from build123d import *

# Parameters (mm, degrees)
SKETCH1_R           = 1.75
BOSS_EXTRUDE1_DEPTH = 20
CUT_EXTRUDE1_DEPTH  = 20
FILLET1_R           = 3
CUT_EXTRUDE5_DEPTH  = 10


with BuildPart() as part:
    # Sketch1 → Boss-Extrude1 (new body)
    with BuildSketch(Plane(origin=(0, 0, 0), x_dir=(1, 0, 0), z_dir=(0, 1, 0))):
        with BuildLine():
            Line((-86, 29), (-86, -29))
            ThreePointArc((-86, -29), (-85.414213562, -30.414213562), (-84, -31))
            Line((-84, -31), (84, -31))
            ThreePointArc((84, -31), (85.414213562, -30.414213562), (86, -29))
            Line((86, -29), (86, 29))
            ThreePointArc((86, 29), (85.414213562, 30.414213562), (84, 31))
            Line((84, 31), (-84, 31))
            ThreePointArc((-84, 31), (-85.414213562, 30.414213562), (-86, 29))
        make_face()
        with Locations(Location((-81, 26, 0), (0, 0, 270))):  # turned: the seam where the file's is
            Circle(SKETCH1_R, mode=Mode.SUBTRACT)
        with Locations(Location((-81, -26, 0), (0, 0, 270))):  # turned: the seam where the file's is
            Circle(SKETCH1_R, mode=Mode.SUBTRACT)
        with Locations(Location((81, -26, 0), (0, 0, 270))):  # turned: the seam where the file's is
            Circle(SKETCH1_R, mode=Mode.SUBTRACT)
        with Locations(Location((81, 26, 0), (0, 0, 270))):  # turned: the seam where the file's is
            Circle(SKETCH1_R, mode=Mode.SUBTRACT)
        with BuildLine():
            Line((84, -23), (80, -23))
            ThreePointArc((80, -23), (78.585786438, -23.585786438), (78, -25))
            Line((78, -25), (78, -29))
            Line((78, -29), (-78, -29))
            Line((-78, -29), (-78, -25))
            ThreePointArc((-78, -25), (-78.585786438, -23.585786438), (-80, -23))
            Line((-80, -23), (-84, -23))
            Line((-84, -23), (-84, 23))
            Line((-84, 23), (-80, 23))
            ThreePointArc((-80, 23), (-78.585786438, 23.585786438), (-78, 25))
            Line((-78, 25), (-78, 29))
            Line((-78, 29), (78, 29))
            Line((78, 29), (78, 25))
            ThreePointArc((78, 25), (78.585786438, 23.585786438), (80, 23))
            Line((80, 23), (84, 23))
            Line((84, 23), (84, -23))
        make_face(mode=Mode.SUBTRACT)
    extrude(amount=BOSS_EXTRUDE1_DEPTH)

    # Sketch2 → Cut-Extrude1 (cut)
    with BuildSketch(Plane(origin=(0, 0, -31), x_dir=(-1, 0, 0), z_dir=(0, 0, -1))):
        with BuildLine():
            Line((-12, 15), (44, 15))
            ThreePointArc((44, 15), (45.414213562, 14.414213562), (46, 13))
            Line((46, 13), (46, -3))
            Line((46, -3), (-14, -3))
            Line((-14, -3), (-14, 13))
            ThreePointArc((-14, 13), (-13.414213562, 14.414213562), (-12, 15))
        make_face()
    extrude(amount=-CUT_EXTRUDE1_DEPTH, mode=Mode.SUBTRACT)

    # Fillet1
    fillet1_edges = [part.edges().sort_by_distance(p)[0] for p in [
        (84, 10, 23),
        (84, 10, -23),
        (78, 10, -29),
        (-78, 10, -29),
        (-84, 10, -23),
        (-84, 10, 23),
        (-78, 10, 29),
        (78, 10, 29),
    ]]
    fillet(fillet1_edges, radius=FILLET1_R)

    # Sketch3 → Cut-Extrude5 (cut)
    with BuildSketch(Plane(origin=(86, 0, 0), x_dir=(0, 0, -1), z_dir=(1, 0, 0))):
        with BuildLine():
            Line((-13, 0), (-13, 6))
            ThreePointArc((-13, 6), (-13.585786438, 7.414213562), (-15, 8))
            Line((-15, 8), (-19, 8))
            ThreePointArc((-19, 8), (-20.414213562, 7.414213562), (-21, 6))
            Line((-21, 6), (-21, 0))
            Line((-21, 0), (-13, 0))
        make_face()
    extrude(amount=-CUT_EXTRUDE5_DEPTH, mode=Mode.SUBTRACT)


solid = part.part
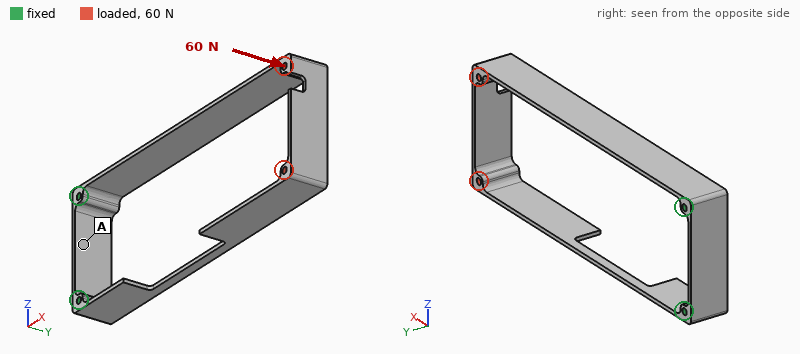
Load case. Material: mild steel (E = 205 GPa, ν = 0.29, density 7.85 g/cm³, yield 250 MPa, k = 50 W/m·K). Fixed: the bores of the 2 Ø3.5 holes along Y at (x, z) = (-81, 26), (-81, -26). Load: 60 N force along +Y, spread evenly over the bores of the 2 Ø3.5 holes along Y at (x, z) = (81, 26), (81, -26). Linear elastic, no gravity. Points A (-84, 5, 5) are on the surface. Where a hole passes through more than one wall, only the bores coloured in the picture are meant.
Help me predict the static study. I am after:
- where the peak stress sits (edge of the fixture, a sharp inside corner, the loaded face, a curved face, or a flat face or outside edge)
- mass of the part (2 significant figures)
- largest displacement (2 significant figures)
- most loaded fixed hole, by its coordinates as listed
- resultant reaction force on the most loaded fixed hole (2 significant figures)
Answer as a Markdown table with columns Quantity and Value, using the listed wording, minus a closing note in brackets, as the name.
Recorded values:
| Quantity | Value |
|---|---|
| where the peak stress sits | a curved face |
| mass of the part | 150 g |
| largest displacement | 1.4 mm |
| most loaded fixed hole, by its coordinates as listed | (-81, 26) |
| resultant reaction force on the most loaded fixed hole | 47 N |
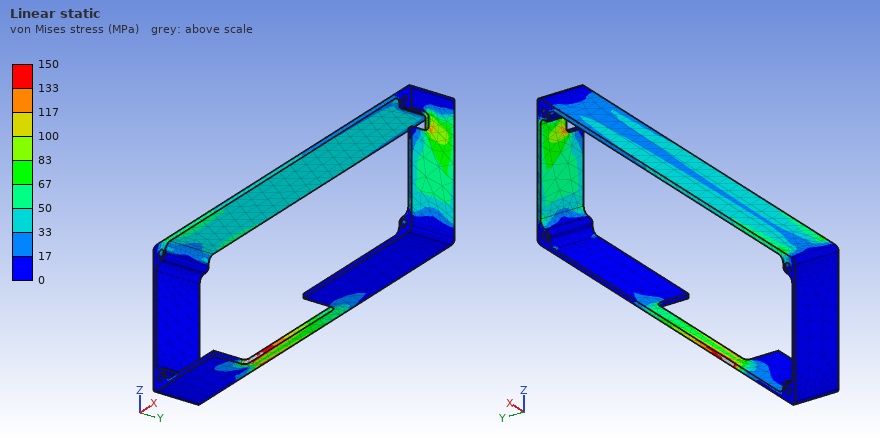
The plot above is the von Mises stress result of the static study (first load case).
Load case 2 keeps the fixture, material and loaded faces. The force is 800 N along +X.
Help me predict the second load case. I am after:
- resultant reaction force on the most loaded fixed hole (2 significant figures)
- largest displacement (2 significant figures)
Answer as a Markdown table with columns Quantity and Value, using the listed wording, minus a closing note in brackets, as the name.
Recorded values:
| Quantity | Value |
|---|---|
| resultant reaction force on the most loaded fixed hole | 400 N |
| largest displacement | 1.2 mm |
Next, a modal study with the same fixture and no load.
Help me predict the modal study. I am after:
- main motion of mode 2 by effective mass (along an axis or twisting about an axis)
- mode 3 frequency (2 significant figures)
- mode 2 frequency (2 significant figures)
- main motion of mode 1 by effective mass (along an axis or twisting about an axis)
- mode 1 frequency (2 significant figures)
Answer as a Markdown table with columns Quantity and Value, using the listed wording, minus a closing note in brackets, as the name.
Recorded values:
| Quantity | Value |
|---|---|
| main motion of mode 2 by effective mass | along Y |
| mode 3 frequency | 350 Hz |
| mode 2 frequency | 160 Hz |
| main motion of mode 1 by effective mass | along Z |
| mode 1 frequency | 74 Hz |
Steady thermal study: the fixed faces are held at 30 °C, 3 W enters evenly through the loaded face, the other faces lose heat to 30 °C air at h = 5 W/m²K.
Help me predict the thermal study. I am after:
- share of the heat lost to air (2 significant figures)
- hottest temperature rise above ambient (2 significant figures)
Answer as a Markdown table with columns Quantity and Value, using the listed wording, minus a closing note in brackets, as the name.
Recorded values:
| Quantity | Value |
|---|---|
| share of the heat lost to air | 78 % |
| hottest temperature rise above ambient | 57 K |
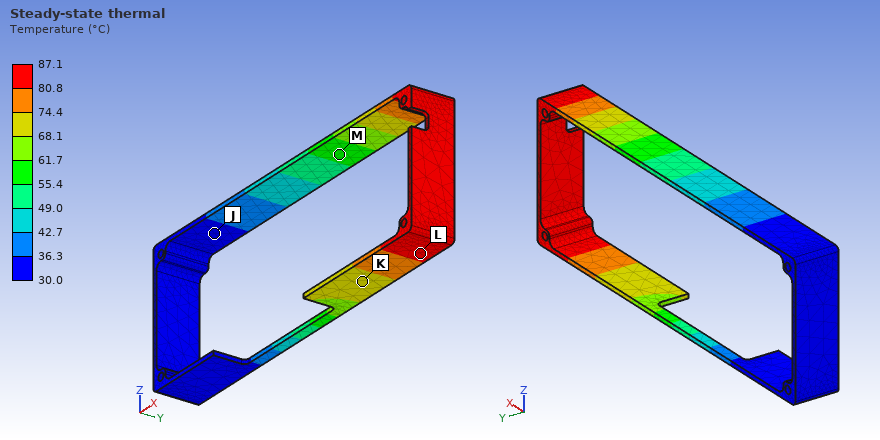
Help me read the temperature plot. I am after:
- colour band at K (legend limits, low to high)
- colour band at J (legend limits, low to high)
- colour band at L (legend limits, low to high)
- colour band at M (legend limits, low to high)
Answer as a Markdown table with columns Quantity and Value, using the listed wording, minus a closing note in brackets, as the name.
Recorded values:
| Quantity | Value |
|---|---|
| colour band at K | 68.1 to 74.4 °C |
| colour band at J | 30.0 to 36.3 °C |
| colour band at L | 80.8 to 87.1 °C |
| colour band at M | 55.4 to 61.7 °C |
